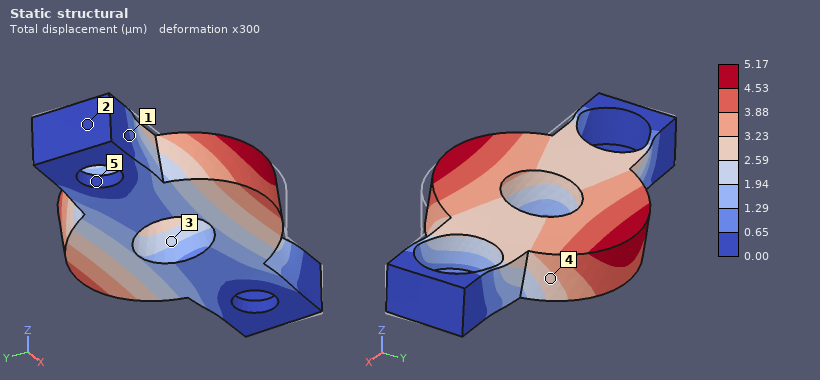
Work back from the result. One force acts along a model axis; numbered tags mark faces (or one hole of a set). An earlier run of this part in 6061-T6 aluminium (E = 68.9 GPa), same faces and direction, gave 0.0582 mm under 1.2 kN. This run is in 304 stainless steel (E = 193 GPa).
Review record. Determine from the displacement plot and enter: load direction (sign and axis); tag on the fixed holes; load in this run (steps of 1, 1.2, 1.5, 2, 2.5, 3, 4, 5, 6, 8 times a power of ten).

+Y
5
300 N
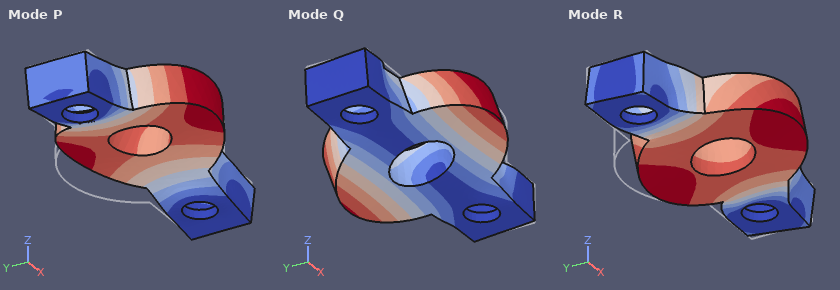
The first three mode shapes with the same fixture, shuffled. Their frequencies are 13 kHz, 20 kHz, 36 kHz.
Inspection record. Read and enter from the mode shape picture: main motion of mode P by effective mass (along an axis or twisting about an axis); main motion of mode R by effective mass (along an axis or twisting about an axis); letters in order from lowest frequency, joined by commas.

along Z
along Y
Q, P, R
